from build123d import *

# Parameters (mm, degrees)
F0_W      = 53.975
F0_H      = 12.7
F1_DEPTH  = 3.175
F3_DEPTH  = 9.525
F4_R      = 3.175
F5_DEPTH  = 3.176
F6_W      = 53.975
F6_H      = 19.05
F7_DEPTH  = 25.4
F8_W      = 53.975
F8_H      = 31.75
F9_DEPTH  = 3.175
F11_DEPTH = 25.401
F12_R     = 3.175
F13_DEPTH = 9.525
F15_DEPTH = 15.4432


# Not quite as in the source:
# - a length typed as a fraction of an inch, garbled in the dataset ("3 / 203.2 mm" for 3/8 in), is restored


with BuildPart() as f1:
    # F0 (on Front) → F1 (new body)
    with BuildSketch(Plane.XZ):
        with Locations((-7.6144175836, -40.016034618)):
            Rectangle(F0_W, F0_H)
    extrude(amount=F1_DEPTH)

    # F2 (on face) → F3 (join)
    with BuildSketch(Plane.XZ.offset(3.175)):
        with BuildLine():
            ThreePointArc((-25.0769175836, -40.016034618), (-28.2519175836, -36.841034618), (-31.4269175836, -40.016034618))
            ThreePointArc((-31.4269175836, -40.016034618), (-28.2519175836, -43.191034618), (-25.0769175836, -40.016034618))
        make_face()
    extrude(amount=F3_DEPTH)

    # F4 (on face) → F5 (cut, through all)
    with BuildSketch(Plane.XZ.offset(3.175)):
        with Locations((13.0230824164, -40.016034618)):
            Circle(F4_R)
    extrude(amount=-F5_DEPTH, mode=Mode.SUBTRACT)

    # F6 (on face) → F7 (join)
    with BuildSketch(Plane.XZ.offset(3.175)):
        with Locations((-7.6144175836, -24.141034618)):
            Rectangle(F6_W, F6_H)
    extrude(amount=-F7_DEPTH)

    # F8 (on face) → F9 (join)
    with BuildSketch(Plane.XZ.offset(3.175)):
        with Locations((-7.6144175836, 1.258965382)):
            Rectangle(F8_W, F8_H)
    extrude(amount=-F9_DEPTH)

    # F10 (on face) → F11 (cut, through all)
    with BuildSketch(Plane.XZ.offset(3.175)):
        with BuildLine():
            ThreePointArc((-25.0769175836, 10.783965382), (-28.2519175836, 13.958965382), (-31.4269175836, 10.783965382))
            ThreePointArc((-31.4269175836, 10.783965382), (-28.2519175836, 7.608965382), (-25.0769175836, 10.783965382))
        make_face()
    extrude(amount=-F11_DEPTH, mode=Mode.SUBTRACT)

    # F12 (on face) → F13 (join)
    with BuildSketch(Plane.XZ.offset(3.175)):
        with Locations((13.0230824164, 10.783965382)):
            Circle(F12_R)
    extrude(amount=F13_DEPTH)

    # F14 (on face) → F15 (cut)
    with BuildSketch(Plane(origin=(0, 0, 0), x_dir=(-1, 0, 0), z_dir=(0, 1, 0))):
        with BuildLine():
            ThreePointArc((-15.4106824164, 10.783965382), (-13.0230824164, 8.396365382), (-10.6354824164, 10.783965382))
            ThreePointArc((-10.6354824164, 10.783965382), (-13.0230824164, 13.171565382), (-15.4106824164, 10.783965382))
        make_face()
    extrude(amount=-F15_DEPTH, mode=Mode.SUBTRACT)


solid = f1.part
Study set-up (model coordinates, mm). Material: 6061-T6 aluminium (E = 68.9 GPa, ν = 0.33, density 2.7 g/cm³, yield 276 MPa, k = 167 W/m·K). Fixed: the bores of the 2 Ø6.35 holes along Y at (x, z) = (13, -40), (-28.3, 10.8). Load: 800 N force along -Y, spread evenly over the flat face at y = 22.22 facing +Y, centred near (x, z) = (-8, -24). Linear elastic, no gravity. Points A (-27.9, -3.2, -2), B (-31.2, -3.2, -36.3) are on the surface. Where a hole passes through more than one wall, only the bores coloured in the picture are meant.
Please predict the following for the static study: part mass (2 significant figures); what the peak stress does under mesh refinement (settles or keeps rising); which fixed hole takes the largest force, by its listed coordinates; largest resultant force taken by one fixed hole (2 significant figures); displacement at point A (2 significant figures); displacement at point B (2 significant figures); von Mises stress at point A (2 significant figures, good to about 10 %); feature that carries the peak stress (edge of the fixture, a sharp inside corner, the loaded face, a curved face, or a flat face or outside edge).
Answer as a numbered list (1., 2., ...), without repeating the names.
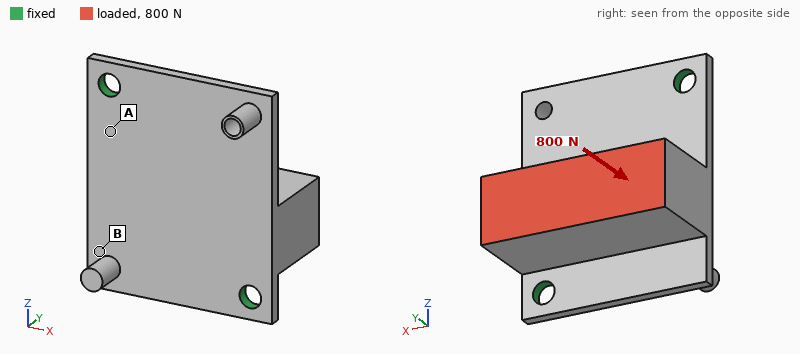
1. 92 g
2. keeps rising
3. (13, -40)
4. 520 N
5. 0.043 mm
6. 0.13 mm
7. 26 MPa
8. edge of the fixture
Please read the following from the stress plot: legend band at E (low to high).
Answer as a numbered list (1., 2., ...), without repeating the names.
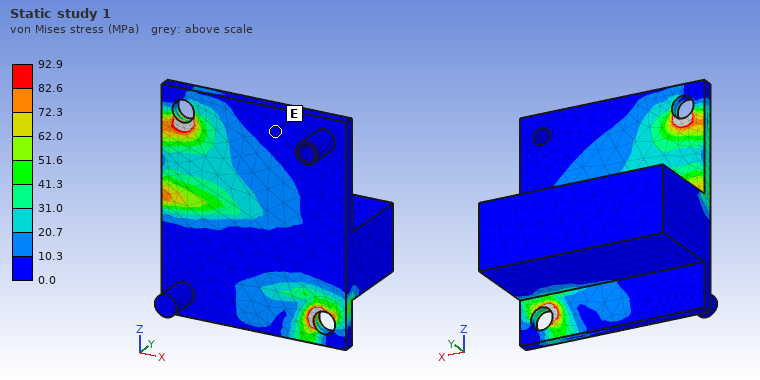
1. 0.0 to 10.3 MPa
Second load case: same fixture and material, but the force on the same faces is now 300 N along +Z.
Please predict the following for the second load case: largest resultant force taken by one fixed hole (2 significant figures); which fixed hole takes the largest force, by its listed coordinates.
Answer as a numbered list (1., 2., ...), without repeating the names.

1. 220 N
2. (13, -40)
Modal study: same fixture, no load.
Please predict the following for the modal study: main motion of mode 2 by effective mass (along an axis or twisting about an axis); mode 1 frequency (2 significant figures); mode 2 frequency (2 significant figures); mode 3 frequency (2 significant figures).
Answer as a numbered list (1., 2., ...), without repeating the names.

1. along Y
2. 1200 Hz
3. 2000 Hz
4. 3700 Hz
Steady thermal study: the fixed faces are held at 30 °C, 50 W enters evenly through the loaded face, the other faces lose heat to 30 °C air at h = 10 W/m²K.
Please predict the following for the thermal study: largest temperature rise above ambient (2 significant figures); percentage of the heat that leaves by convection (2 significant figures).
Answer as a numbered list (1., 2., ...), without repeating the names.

1. 35 K
2. 4.8 %
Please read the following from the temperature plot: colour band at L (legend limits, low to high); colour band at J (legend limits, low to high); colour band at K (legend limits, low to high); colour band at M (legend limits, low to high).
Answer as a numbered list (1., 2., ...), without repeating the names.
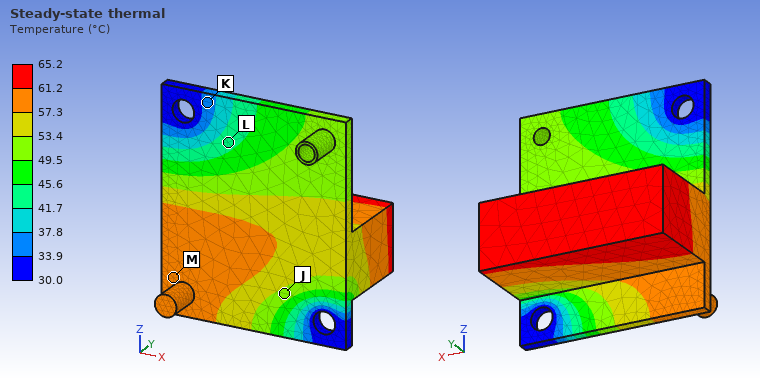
1. 41.7 to 45.6 °C
2. 49.5 to 53.4 °C
3. 33.9 to 37.8 °C
4. 57.3 to 61.2 °C
